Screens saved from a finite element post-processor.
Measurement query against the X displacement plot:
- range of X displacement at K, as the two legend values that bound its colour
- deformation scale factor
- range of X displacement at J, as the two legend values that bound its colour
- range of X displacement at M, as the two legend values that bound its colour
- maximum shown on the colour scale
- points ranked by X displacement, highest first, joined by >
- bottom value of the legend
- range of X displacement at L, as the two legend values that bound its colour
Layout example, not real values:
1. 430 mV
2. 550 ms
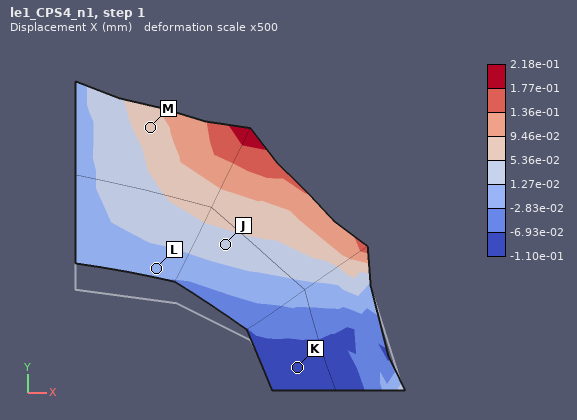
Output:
1. -1.10e-01 to -6.93e-02 mm
2. 500
3. 1.27e-02 to 5.36e-02 mm
4. 5.36e-02 to 9.46e-02 mm
5. 2.18e-01 mm
6. M > J > L > K
7. -1.10e-01 mm
8. -2.83e-02 to 1.27e-02 mm
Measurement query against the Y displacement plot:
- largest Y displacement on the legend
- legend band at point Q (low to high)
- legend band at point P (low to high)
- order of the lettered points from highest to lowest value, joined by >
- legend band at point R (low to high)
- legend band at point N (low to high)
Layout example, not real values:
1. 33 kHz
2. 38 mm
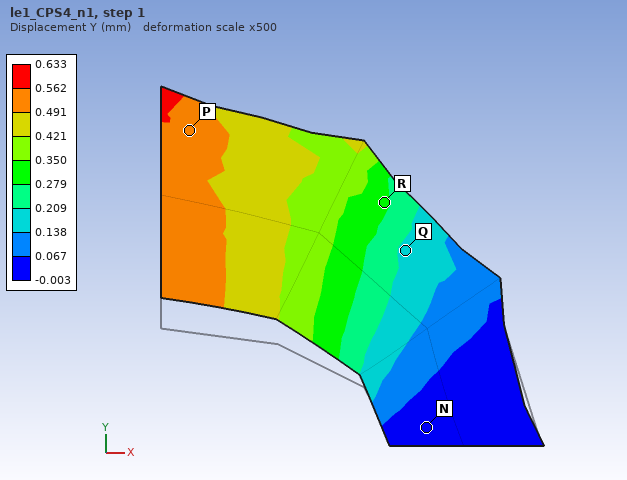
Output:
1. 0.633 mm
2. 0.138 to 0.209 mm
3. 0.491 to 0.562 mm
4. P > R > Q > N
5. 0.279 to 0.350 mm
6. -0.003 to 0.067 mm
